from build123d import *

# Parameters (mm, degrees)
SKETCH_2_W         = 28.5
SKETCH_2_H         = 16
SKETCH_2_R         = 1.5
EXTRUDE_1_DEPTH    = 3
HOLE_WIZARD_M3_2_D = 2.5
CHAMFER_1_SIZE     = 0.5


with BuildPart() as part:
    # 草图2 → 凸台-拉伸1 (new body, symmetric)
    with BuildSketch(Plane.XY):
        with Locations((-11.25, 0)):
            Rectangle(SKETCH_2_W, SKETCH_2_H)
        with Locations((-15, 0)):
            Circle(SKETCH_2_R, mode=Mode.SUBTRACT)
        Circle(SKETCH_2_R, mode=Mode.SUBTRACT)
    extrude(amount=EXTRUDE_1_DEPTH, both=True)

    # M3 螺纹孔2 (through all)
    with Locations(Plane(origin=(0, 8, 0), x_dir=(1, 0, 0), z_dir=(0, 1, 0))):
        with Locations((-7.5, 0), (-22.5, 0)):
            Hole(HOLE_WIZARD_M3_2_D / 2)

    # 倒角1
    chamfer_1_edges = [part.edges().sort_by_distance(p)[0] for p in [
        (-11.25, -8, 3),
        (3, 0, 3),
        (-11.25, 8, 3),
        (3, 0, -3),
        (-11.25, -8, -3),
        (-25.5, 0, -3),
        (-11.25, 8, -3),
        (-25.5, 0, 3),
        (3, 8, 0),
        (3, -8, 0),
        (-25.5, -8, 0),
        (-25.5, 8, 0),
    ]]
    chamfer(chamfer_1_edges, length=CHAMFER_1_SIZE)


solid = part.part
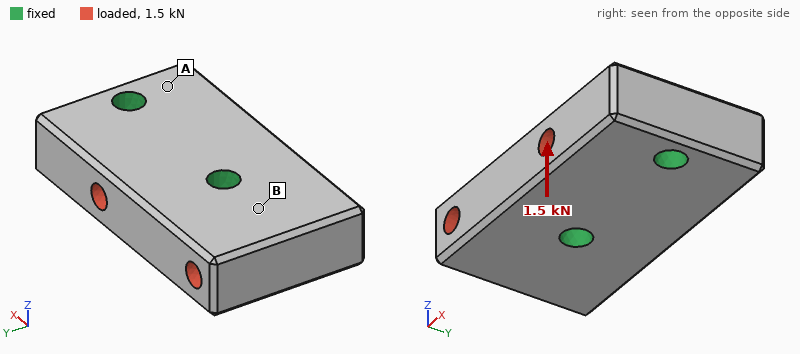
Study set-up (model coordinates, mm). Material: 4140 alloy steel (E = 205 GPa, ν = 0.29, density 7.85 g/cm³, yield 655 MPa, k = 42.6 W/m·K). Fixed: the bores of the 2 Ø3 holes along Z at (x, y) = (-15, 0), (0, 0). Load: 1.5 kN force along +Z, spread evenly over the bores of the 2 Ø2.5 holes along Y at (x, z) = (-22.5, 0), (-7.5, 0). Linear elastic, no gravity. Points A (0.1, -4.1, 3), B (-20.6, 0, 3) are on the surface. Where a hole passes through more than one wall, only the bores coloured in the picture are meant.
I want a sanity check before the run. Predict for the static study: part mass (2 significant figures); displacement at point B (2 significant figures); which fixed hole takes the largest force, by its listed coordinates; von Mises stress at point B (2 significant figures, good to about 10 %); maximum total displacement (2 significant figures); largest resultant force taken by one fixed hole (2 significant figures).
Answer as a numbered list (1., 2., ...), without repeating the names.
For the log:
1. 19 g
2. 2.3 µm
3. (-15, 0)
4. 24 MPa
5. 4.9 µm
6. 1.2 kN
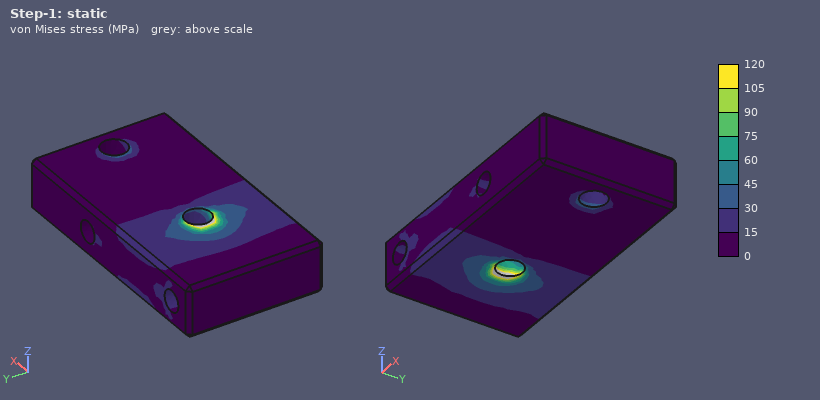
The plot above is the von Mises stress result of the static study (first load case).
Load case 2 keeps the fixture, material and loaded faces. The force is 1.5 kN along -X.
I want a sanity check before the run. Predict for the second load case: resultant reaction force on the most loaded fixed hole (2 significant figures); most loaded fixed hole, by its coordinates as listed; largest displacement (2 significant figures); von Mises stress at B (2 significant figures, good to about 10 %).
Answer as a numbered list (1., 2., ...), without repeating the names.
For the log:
1. 1.0 kN
2. (-15, 0)
3. 0.71 µm
4. 12 MPa
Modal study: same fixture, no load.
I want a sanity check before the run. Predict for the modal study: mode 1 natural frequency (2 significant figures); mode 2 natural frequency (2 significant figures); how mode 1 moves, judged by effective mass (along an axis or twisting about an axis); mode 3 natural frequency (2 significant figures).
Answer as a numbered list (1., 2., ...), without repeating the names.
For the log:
1. 34 kHz
2. 41 kHz
3. along Z
4. 42 kHz
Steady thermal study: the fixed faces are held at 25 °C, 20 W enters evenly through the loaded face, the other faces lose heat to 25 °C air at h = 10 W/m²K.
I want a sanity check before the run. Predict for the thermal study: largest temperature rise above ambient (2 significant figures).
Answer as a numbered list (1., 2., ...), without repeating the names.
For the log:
1. 27 K
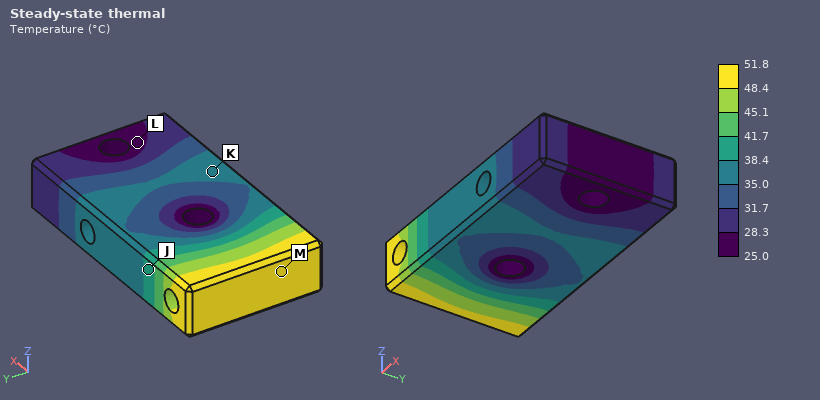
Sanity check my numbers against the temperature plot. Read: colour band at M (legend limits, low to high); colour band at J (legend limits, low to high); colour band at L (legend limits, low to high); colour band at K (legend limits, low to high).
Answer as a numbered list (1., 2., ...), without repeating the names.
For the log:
1. 48.4 to 51.8 °C
2. 38.4 to 41.7 °C
3. 25.0 to 28.3 °C
4. 35.0 to 38.4 °C
